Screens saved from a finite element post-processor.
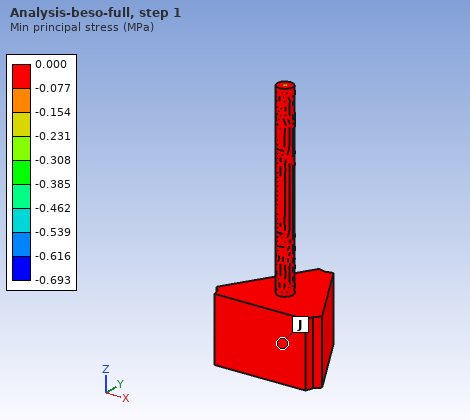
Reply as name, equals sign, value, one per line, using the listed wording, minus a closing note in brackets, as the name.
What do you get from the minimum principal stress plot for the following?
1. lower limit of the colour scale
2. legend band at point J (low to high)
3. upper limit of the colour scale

lower limit of the colour scale = -0.693 MPa
legend band at point J = -0.077 to 0.000 MPa
upper limit of the colour scale = 0.000 MPa
